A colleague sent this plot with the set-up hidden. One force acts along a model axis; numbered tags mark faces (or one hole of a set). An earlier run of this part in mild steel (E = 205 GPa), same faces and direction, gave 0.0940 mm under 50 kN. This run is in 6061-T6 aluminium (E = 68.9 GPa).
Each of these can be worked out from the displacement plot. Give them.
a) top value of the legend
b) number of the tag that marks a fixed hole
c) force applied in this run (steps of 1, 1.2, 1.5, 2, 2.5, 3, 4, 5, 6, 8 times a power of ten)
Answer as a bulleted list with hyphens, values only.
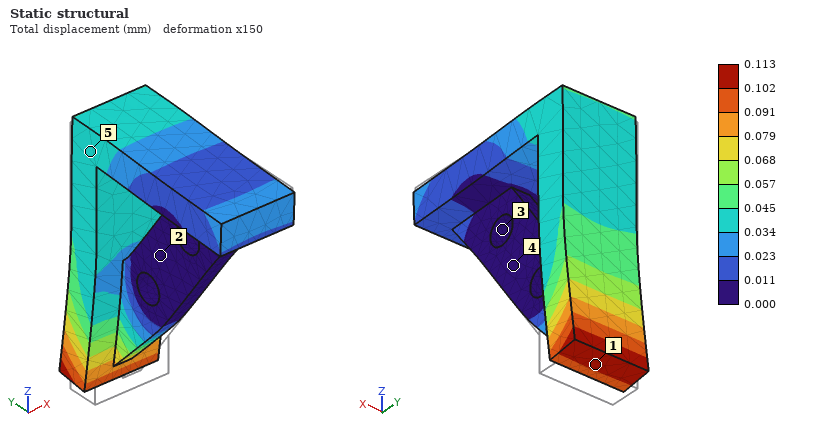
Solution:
- 0.113 mm
- 3
- 20 kN
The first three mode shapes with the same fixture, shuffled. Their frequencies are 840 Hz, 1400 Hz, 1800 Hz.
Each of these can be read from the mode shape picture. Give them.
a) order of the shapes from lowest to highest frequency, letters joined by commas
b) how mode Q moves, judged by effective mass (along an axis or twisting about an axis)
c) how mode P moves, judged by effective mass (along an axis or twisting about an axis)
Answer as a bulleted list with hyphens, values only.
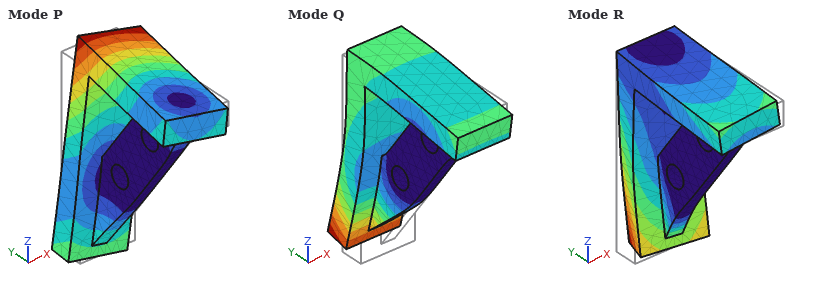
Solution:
- P, R, Q
- along Z
- along X
